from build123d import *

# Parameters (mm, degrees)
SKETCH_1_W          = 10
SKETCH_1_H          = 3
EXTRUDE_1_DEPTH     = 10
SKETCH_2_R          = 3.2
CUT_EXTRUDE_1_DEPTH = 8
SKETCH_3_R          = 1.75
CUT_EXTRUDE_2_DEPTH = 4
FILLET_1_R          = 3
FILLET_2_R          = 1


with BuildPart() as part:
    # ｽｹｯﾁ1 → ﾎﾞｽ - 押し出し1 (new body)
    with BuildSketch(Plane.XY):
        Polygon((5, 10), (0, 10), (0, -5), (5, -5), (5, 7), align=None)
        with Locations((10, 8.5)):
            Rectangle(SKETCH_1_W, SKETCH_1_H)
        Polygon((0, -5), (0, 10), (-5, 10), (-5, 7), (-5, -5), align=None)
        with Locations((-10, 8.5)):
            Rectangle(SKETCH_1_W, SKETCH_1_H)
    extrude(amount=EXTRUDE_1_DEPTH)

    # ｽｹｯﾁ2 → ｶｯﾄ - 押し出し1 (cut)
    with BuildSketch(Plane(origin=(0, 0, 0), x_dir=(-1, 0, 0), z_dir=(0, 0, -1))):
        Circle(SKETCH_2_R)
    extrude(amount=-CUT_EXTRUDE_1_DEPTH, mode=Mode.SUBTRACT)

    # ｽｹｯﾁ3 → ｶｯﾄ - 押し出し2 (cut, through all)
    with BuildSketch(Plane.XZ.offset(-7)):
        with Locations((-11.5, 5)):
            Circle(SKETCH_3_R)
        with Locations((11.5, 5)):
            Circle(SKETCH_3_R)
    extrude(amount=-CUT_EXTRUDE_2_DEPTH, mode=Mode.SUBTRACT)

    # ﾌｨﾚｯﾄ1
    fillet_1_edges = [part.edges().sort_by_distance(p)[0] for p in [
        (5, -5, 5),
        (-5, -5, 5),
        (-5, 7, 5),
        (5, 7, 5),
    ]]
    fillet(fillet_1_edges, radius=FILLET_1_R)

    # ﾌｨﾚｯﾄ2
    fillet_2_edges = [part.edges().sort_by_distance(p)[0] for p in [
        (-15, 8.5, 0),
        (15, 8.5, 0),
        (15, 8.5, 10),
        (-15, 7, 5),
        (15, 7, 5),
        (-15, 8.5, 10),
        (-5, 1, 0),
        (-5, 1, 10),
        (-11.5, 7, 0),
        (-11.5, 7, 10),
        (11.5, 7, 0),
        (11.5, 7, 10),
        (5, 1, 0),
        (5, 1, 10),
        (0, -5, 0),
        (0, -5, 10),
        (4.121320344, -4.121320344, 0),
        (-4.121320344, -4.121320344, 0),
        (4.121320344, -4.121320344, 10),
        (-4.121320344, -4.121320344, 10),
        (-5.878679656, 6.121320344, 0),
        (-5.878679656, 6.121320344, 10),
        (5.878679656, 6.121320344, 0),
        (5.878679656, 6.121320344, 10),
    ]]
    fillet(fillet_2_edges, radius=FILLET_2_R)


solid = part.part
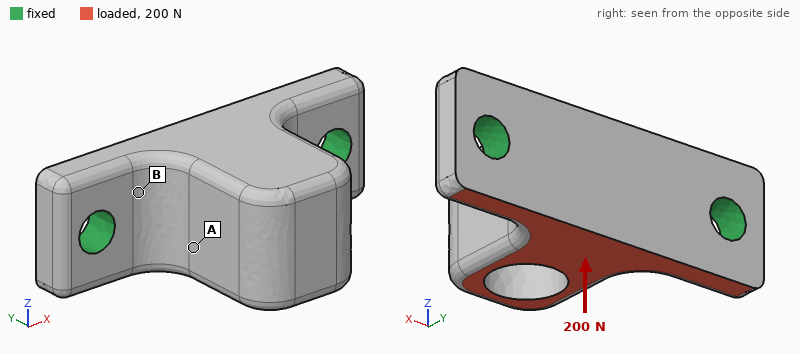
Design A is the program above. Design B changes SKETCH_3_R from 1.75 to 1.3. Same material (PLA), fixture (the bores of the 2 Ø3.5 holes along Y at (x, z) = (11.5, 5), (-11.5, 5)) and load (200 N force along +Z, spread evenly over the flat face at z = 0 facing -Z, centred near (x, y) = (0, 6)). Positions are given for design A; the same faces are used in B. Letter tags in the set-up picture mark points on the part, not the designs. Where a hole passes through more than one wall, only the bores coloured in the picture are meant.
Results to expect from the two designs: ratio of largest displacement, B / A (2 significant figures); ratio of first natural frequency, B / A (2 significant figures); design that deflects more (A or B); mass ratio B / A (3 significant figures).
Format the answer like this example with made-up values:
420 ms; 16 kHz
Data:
1.2; 0.91; B; 1.01
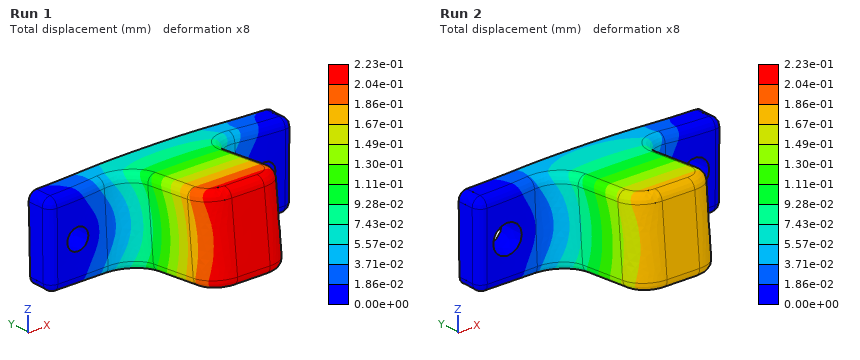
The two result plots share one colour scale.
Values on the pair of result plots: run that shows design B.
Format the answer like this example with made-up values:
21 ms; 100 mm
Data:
Run 1
